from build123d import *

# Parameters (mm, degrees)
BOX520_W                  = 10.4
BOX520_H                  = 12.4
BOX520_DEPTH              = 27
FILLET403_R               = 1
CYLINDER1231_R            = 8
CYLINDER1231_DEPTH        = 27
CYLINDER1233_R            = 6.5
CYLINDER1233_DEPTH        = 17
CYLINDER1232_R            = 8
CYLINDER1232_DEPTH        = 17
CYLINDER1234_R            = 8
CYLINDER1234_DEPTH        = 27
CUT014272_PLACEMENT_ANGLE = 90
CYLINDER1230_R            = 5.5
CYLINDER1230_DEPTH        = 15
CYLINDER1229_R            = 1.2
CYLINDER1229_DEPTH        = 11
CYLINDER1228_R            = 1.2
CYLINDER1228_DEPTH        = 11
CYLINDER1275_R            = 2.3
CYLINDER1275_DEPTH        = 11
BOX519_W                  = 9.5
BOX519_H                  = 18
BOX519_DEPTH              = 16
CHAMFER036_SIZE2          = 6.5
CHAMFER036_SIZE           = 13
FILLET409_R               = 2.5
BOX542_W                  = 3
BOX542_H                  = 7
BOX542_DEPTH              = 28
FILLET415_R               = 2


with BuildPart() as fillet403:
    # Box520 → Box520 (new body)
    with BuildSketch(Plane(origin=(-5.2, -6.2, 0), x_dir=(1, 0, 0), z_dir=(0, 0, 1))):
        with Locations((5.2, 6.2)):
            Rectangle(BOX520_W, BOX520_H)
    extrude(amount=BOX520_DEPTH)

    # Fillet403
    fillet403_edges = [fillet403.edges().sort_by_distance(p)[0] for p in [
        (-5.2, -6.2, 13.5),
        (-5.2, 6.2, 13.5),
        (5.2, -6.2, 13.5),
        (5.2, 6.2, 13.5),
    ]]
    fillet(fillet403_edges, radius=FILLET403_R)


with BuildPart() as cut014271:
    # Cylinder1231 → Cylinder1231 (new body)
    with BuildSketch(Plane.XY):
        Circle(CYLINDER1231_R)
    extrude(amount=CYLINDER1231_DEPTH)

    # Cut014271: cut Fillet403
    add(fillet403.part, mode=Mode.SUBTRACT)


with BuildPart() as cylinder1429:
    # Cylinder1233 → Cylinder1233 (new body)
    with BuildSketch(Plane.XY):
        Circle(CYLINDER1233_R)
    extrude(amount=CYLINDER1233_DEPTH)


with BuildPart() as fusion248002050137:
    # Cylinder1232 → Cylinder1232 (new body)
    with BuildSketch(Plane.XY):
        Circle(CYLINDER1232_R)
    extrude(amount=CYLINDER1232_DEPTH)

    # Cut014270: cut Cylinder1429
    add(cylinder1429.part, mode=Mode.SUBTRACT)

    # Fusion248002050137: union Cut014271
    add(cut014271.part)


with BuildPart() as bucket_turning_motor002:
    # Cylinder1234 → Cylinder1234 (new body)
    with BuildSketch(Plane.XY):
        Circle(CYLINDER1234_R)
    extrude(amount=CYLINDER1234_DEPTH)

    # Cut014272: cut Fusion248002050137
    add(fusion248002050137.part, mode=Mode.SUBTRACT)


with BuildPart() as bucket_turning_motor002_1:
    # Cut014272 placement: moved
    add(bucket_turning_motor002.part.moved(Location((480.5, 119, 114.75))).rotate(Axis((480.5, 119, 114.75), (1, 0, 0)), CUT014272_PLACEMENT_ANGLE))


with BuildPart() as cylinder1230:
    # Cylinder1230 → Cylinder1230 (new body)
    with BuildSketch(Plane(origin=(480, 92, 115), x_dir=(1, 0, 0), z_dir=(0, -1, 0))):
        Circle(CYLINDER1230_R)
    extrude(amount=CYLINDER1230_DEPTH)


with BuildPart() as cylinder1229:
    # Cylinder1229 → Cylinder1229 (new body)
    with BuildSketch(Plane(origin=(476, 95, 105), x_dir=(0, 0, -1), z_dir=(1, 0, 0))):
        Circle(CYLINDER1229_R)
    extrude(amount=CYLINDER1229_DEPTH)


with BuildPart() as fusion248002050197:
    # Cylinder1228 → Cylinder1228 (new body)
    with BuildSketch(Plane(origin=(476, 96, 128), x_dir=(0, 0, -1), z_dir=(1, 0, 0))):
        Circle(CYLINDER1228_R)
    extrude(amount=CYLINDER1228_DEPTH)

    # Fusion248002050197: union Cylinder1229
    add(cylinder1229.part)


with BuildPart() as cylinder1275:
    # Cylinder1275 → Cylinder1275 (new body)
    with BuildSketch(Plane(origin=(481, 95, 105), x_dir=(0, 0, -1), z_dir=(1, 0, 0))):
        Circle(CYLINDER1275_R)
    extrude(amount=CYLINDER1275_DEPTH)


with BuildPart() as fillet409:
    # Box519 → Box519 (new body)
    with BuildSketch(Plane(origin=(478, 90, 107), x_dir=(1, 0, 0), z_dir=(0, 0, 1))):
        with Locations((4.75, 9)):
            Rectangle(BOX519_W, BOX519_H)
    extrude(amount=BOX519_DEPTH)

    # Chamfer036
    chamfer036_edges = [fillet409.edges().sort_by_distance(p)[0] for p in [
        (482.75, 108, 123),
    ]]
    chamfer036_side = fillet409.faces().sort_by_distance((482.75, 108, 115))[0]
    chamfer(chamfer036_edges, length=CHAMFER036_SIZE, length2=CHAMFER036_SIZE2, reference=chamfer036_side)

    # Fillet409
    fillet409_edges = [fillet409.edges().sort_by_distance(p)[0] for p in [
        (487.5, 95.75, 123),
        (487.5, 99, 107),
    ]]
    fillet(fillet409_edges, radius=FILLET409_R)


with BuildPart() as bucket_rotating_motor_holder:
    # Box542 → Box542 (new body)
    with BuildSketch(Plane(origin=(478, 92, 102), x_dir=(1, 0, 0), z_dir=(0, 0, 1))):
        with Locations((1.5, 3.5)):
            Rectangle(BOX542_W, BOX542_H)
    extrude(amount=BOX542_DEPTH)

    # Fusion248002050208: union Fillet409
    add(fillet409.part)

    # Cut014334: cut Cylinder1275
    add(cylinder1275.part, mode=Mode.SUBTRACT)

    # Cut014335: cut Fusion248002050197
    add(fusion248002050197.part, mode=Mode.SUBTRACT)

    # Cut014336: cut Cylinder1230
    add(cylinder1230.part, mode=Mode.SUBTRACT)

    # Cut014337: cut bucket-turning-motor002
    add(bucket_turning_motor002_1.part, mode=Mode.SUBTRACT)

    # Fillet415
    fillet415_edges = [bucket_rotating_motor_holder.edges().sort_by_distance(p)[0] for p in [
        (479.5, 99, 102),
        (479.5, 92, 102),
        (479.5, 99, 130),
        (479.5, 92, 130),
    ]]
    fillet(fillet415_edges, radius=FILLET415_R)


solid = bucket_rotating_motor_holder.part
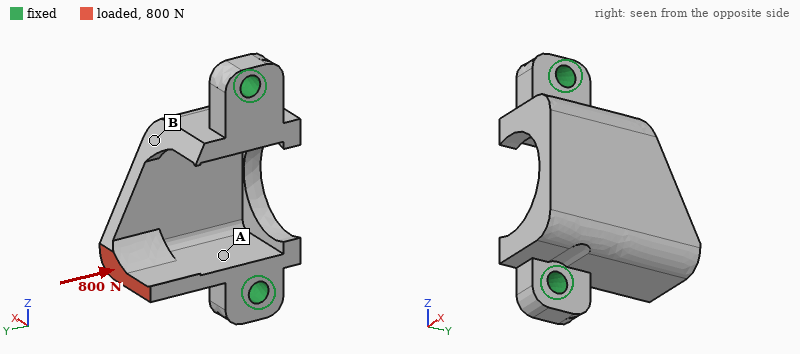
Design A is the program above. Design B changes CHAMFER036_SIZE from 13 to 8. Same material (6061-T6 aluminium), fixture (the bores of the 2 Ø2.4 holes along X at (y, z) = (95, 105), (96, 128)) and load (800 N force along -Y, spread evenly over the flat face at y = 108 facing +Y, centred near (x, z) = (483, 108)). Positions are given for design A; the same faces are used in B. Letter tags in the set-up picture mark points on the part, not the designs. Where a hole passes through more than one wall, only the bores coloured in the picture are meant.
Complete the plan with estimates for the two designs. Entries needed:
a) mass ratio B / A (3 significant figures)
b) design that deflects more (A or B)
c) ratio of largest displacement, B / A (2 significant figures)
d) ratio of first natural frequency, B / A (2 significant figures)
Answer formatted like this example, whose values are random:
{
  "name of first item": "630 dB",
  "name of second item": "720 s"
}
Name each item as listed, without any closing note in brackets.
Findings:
{
  "mass ratio B / A": "1.03",
  "design that deflects more": "B",
  "ratio of largest displacement, B / A": "1.2",
  "ratio of first natural frequency, B / A": "0.95"
}
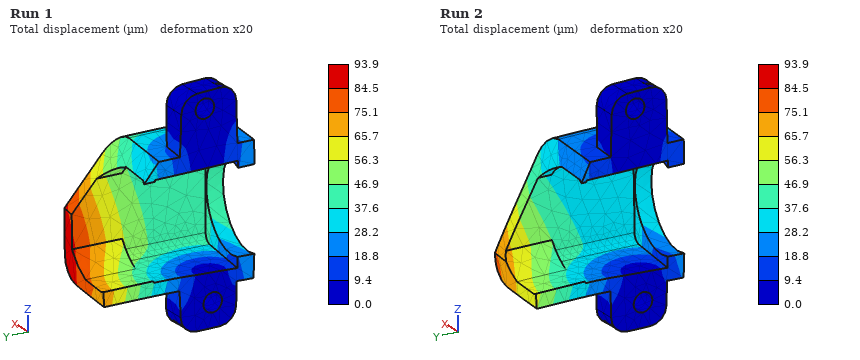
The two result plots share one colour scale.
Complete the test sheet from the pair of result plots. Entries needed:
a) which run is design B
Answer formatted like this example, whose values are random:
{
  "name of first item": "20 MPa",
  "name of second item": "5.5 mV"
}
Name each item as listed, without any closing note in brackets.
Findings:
{
  "which run is design B": "Run 1"
}
